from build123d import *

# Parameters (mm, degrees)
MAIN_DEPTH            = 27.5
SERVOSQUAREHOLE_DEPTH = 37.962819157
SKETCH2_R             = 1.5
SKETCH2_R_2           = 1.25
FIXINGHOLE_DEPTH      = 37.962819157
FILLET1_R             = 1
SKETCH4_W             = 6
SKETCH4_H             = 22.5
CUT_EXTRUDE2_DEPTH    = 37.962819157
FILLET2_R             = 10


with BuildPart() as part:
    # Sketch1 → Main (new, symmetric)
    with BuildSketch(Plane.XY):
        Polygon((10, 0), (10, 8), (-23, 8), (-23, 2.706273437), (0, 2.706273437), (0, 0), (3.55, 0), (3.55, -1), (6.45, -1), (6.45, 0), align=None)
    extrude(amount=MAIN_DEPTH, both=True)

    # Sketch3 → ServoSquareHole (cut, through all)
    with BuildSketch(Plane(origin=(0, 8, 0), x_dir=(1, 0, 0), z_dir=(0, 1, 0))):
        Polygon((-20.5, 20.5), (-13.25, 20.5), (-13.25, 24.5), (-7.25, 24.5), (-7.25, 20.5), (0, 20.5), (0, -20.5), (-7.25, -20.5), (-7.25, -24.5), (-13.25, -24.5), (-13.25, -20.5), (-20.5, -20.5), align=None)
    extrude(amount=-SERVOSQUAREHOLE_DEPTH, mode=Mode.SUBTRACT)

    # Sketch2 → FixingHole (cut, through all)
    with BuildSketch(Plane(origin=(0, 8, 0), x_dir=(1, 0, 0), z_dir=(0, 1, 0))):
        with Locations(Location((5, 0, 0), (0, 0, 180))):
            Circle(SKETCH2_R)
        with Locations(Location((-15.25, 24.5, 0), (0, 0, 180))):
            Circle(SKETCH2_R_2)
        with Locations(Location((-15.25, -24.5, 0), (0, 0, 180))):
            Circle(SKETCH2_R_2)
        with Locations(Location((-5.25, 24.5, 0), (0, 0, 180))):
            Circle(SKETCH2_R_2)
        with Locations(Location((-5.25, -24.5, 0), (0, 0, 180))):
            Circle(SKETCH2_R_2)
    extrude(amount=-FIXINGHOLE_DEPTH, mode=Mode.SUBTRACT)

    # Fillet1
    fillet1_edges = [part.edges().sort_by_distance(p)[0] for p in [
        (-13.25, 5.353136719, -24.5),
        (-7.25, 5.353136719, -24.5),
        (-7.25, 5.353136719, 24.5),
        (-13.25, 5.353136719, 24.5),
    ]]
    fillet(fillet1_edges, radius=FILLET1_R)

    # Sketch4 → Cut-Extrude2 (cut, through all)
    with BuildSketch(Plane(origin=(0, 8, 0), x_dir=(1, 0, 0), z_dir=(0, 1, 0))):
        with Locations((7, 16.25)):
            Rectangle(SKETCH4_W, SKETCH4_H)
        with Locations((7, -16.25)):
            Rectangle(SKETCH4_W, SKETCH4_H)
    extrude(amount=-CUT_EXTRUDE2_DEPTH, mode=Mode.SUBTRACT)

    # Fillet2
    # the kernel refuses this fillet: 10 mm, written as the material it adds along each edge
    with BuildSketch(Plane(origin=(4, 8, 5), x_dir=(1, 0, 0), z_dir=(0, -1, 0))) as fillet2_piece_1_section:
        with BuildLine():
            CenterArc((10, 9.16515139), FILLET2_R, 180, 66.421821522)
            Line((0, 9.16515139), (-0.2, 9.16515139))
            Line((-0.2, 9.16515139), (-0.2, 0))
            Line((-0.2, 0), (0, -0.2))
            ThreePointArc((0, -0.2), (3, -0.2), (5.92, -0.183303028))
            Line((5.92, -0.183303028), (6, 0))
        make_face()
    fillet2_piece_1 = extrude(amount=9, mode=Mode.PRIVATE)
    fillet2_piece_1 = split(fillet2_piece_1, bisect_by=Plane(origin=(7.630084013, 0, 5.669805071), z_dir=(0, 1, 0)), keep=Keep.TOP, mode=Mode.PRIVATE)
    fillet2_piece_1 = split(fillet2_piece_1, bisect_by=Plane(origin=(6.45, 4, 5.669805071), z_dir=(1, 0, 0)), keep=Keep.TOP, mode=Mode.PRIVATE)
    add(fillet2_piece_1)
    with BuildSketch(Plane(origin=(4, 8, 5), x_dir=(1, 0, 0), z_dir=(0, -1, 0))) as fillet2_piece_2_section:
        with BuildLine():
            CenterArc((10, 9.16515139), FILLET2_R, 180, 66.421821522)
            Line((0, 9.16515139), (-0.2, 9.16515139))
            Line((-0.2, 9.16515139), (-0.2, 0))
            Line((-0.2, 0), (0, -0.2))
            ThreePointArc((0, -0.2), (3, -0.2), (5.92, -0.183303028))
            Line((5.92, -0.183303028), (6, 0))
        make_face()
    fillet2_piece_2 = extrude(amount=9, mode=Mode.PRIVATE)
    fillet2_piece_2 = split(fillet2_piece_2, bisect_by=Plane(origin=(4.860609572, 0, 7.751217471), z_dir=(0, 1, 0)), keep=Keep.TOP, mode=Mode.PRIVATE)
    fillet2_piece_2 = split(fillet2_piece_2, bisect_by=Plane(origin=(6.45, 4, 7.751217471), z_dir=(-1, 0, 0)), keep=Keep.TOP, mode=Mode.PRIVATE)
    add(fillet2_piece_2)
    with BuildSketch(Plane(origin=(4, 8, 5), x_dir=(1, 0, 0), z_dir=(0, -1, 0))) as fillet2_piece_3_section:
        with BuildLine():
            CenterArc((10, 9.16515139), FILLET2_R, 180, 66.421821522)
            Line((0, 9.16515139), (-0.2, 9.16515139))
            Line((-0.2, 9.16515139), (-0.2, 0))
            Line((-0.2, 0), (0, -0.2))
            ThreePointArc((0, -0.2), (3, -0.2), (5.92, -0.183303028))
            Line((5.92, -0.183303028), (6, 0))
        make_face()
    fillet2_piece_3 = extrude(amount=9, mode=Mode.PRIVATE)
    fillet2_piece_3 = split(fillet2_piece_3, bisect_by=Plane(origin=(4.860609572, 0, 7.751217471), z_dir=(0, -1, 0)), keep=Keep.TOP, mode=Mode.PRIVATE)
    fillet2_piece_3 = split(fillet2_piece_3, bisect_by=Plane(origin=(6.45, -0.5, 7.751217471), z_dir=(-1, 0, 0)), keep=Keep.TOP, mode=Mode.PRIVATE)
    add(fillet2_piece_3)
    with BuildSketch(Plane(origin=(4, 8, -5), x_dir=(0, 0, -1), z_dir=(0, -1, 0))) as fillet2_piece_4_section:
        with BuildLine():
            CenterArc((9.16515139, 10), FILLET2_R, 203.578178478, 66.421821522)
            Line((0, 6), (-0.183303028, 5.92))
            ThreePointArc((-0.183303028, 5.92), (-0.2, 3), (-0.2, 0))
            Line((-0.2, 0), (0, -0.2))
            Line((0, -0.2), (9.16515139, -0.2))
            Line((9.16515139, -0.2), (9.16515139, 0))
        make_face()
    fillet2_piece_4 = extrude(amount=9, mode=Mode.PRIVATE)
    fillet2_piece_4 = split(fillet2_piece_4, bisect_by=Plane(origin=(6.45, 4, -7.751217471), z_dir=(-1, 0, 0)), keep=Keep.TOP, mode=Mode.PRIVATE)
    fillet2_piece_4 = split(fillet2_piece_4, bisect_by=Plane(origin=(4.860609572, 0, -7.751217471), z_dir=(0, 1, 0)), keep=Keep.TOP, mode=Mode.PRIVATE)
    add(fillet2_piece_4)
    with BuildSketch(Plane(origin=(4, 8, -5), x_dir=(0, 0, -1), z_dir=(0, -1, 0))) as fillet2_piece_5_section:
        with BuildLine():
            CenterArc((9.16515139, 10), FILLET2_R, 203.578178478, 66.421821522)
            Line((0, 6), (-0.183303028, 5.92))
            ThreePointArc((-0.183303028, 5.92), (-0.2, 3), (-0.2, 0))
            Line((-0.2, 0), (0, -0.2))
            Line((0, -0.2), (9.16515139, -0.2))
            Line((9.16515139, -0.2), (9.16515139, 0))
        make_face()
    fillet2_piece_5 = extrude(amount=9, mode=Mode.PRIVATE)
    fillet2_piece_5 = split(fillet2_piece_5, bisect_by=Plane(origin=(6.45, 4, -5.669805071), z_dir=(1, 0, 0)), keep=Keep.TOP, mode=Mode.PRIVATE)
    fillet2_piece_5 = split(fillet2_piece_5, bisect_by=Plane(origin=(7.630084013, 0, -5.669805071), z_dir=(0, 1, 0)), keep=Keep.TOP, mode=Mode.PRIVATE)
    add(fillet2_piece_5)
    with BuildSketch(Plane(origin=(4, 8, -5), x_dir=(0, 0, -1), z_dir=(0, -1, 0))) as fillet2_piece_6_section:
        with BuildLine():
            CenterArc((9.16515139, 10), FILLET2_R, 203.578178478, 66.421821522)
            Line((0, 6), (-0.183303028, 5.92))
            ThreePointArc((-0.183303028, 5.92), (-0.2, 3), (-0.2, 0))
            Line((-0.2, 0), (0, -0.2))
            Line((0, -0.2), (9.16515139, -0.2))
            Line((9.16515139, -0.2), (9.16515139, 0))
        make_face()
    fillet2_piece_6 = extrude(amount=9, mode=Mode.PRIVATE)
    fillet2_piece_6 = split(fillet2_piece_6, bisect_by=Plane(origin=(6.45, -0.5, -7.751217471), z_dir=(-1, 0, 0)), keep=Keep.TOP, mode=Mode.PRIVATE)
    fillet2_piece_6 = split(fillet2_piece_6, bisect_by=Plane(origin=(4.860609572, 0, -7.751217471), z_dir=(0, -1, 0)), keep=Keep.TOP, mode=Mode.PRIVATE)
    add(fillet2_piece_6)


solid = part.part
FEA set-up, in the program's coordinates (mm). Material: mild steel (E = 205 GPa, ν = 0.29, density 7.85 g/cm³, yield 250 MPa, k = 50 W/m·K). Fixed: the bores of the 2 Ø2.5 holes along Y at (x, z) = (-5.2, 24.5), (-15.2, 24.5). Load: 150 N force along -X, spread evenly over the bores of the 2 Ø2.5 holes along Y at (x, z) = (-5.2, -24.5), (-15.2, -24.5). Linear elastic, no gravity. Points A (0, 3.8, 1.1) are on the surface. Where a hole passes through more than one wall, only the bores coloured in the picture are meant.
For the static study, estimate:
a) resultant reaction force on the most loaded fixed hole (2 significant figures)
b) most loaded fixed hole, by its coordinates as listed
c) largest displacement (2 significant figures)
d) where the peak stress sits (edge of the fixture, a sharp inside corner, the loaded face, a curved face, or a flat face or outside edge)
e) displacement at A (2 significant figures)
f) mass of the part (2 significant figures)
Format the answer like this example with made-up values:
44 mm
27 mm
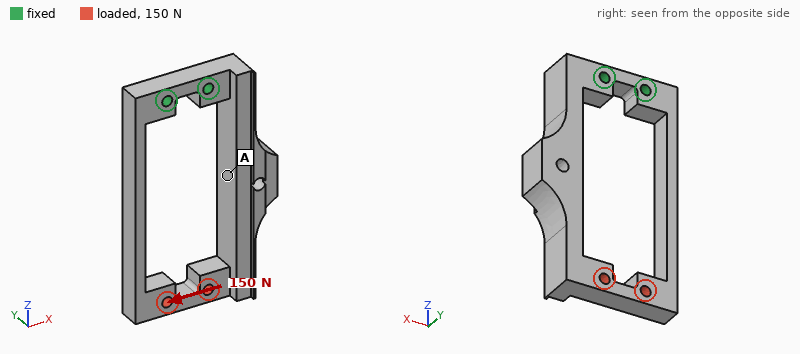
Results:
280 N
(-5.2, 24.5)
0.18 mm
a curved face
0.077 mm
34 g
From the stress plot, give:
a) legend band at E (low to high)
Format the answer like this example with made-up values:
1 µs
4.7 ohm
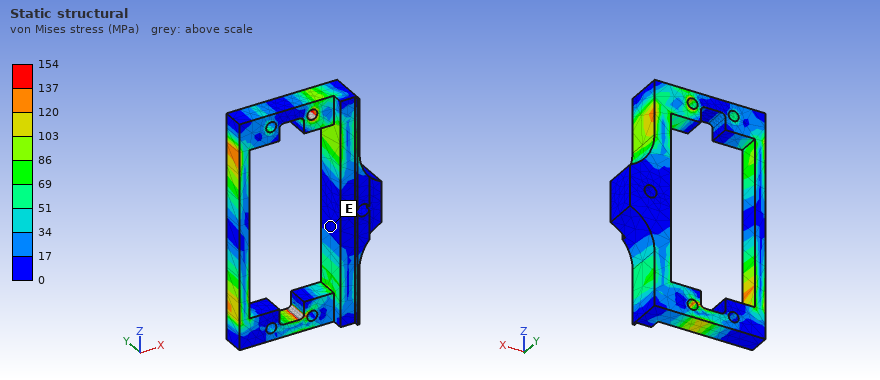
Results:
0 to 17 MPa
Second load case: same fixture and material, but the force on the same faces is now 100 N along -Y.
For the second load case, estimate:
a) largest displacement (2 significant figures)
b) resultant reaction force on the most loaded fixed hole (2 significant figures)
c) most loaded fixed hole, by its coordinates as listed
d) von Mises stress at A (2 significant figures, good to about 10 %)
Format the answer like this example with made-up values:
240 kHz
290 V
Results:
0.18 mm
66 N
(-5.2, 24.5)
11 MPa
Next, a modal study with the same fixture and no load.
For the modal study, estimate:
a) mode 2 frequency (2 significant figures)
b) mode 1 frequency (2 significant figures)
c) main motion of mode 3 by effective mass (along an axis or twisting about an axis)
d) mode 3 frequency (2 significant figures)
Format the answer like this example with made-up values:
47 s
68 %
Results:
1300 Hz
1200 Hz
twisting about Z
2900 Hz
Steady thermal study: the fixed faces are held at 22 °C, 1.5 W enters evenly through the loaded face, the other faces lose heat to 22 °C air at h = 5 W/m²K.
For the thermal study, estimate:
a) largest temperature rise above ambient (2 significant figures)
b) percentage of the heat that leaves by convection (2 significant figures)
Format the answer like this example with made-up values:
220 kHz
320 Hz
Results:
31 K
16 %
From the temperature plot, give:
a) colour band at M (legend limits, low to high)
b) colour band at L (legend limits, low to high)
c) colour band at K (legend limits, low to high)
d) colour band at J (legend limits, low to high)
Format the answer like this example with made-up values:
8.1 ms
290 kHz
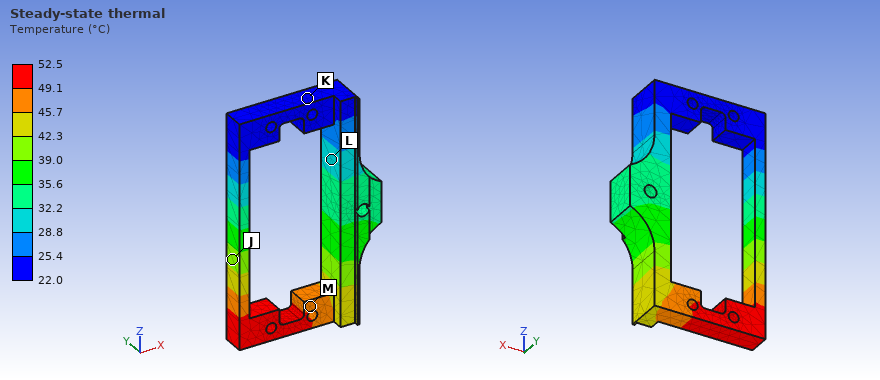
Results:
45.7 to 49.1 °C
28.8 to 32.2 °C
22.0 to 25.4 °C
39.0 to 42.3 °C
